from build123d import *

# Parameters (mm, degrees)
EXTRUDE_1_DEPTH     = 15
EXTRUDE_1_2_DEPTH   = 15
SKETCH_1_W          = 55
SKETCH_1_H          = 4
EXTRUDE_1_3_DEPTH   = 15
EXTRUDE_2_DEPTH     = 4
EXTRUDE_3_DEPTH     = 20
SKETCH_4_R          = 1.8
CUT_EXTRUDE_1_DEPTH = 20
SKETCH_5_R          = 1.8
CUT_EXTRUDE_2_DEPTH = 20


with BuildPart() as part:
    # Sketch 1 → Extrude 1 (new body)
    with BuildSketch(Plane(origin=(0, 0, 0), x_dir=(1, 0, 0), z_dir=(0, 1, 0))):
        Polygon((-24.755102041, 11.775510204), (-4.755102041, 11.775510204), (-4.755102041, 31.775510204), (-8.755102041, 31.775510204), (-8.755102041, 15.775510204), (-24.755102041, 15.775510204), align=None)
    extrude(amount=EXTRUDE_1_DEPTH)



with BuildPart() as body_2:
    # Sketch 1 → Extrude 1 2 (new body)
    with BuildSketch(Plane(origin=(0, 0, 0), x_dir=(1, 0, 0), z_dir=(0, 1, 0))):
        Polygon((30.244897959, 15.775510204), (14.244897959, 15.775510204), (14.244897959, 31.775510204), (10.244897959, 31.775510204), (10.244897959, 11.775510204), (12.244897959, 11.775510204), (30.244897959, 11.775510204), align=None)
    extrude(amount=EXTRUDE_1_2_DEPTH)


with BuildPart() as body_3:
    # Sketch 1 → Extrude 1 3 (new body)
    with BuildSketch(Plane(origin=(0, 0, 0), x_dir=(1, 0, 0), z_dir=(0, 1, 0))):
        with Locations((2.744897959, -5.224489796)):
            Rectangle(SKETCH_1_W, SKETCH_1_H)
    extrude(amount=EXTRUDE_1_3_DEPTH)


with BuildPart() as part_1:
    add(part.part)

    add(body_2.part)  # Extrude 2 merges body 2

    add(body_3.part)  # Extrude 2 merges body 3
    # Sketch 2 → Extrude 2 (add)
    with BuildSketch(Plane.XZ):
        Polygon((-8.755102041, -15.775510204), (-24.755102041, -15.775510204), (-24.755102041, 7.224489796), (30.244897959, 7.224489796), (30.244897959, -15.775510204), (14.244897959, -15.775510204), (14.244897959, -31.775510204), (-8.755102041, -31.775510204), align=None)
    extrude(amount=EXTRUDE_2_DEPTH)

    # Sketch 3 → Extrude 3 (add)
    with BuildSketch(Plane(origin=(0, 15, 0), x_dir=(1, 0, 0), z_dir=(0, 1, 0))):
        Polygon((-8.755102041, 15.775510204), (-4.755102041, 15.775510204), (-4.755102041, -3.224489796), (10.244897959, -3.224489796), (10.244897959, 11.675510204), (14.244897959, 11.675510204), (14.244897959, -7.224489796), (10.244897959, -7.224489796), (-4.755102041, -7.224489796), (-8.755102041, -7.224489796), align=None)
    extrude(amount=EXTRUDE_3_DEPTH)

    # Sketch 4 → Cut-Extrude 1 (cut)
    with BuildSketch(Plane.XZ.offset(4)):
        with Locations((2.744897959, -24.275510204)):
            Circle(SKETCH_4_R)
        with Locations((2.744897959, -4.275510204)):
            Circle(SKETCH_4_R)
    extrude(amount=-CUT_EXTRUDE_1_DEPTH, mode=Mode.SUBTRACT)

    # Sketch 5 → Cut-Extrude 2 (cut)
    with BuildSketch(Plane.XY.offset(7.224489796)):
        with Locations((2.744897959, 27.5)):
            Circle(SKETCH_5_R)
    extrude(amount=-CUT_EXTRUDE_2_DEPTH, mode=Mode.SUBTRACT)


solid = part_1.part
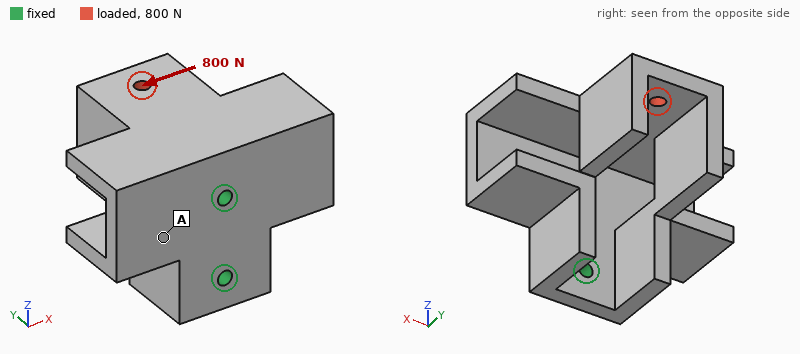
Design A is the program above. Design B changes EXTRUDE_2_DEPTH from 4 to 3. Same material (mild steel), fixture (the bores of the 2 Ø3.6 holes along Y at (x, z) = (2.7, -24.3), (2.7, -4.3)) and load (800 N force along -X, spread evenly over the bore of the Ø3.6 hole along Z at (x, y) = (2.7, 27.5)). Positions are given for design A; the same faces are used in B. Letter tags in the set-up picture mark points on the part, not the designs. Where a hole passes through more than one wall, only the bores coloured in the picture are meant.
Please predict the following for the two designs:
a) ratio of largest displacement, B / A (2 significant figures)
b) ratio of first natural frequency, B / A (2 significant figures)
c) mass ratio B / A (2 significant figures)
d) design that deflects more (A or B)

1.7
0.75
0.91
B
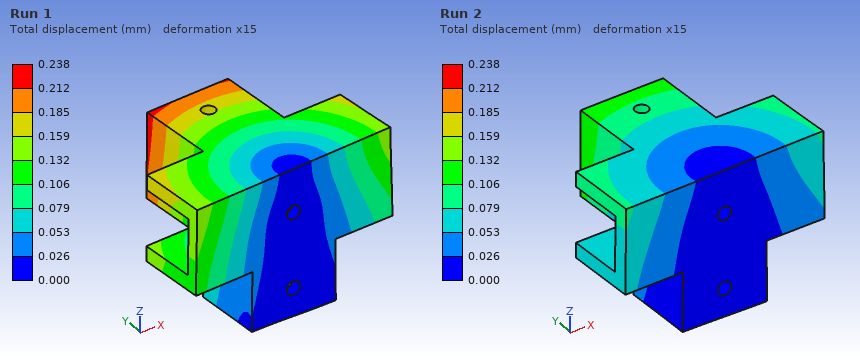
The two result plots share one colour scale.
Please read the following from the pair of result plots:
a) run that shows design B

Run 1
